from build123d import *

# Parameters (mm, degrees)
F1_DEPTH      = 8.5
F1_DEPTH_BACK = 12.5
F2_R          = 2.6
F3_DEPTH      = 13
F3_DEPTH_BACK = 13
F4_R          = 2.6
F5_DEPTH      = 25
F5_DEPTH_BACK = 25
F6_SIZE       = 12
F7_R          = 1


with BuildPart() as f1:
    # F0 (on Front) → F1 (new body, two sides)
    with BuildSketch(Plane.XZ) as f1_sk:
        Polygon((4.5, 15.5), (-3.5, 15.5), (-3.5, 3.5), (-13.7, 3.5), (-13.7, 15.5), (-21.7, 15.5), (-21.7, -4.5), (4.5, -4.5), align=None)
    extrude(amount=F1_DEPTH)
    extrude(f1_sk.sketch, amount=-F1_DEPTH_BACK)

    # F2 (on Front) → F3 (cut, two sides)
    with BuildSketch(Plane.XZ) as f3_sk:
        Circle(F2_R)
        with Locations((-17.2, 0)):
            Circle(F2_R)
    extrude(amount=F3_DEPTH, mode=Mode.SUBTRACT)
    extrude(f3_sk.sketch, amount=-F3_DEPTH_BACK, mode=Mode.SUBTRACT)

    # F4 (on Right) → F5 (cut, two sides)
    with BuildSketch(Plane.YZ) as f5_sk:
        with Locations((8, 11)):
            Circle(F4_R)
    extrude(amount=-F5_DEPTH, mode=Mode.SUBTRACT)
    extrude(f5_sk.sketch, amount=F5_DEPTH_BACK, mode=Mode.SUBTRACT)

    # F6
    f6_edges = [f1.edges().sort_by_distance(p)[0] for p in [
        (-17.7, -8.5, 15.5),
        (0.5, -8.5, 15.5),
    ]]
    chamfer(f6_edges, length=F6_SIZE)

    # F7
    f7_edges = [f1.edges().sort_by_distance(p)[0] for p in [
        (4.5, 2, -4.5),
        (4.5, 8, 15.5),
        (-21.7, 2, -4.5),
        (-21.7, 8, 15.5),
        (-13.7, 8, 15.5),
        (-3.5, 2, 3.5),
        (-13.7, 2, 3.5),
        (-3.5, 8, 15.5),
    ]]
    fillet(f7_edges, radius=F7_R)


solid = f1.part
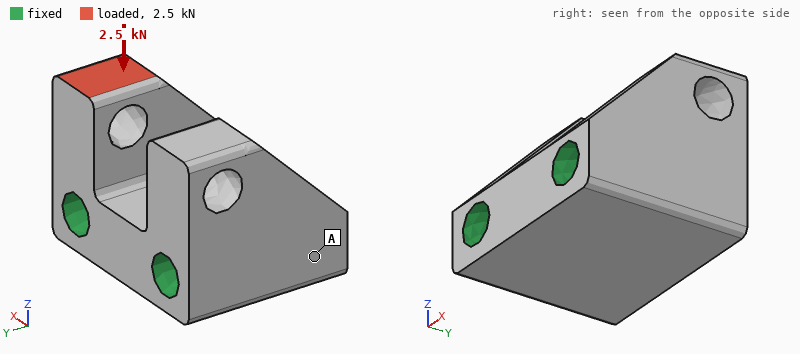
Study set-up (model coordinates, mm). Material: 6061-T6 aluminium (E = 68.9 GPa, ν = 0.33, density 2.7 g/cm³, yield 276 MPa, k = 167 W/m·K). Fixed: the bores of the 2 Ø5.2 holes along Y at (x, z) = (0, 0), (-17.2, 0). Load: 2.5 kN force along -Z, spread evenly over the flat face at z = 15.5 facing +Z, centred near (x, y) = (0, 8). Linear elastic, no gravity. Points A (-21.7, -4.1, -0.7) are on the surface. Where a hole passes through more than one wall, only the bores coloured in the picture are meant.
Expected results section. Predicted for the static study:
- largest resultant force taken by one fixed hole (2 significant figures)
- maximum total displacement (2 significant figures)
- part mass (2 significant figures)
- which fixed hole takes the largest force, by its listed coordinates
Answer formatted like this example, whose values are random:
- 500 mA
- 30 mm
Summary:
- 2.5 kN
- 19 µm
- 16 g
- (0, 0)
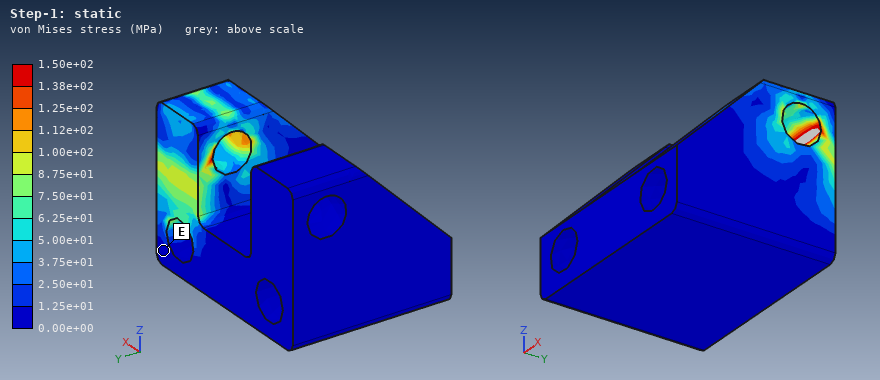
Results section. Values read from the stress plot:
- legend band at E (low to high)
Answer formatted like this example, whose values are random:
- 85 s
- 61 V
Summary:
- 0.00e+00 to 1.25e+01 MPa
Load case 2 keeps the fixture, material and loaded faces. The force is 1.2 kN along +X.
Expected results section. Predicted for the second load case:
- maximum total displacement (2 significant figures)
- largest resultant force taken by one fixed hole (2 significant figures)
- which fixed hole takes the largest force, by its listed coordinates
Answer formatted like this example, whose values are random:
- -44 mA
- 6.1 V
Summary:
- 47 µm
- 980 N
- (0, 0)
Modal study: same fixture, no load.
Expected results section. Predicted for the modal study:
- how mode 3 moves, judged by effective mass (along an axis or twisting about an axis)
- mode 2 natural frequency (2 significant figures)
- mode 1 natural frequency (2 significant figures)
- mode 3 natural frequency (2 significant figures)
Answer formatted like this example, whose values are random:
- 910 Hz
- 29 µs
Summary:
- along Y
- 34 kHz
- 33 kHz
- 51 kHz
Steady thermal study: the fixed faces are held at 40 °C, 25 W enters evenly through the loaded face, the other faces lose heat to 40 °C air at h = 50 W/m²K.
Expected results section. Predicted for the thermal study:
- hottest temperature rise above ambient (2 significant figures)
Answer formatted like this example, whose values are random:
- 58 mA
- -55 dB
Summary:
- 31 K
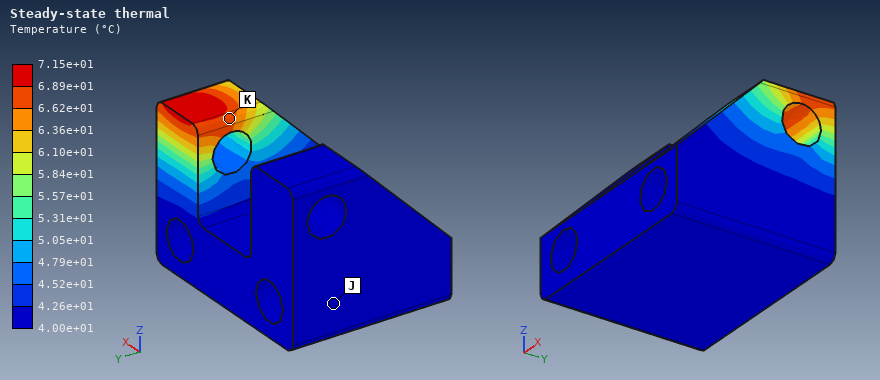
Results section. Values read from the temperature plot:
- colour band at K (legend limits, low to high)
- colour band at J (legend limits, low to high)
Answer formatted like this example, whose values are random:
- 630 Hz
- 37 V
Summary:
- 6.62e+01 to 6.89e+01 °C
- 4.00e+01 to 4.26e+01 °C
